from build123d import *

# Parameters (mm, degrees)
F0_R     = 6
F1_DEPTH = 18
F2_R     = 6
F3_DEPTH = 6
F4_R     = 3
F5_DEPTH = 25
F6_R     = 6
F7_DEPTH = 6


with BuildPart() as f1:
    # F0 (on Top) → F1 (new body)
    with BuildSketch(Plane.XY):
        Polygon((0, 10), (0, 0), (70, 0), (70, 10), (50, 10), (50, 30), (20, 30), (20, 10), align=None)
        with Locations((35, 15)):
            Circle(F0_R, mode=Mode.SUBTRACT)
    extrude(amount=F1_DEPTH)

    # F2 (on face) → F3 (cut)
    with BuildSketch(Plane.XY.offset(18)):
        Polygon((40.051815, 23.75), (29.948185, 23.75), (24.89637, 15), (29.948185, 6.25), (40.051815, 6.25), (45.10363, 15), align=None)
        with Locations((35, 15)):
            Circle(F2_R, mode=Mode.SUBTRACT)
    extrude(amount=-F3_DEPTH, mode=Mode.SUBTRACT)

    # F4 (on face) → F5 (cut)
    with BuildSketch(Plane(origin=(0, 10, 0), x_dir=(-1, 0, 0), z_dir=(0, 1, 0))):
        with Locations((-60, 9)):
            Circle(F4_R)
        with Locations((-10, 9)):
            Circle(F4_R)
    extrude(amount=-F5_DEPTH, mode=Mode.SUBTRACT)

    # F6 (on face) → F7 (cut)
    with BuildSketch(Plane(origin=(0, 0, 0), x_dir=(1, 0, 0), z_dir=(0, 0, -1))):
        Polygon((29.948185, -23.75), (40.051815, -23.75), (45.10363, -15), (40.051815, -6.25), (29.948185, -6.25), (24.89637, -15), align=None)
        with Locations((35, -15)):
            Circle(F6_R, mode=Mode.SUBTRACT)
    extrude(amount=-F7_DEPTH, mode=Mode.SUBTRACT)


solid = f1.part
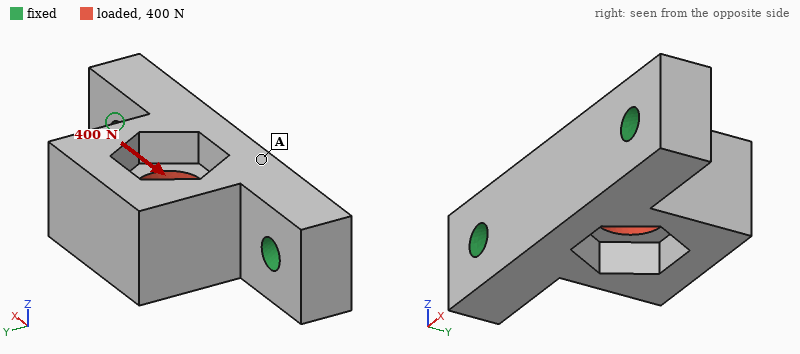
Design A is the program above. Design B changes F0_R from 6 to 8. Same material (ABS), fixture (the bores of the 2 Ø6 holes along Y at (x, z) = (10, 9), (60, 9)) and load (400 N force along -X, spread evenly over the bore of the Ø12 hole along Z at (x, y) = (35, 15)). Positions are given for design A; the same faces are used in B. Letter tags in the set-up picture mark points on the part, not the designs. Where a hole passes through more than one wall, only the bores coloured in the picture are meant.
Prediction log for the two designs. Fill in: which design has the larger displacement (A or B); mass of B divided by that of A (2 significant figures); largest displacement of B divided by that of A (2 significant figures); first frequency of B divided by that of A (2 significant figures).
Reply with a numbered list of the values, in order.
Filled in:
1. B
2. 0.97
3. 1.2
4. 1.0
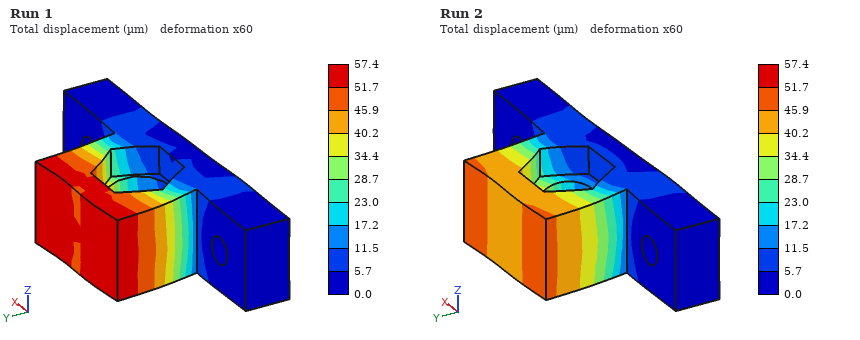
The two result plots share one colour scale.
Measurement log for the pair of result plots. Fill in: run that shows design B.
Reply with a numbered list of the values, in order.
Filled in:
1. Run 1
